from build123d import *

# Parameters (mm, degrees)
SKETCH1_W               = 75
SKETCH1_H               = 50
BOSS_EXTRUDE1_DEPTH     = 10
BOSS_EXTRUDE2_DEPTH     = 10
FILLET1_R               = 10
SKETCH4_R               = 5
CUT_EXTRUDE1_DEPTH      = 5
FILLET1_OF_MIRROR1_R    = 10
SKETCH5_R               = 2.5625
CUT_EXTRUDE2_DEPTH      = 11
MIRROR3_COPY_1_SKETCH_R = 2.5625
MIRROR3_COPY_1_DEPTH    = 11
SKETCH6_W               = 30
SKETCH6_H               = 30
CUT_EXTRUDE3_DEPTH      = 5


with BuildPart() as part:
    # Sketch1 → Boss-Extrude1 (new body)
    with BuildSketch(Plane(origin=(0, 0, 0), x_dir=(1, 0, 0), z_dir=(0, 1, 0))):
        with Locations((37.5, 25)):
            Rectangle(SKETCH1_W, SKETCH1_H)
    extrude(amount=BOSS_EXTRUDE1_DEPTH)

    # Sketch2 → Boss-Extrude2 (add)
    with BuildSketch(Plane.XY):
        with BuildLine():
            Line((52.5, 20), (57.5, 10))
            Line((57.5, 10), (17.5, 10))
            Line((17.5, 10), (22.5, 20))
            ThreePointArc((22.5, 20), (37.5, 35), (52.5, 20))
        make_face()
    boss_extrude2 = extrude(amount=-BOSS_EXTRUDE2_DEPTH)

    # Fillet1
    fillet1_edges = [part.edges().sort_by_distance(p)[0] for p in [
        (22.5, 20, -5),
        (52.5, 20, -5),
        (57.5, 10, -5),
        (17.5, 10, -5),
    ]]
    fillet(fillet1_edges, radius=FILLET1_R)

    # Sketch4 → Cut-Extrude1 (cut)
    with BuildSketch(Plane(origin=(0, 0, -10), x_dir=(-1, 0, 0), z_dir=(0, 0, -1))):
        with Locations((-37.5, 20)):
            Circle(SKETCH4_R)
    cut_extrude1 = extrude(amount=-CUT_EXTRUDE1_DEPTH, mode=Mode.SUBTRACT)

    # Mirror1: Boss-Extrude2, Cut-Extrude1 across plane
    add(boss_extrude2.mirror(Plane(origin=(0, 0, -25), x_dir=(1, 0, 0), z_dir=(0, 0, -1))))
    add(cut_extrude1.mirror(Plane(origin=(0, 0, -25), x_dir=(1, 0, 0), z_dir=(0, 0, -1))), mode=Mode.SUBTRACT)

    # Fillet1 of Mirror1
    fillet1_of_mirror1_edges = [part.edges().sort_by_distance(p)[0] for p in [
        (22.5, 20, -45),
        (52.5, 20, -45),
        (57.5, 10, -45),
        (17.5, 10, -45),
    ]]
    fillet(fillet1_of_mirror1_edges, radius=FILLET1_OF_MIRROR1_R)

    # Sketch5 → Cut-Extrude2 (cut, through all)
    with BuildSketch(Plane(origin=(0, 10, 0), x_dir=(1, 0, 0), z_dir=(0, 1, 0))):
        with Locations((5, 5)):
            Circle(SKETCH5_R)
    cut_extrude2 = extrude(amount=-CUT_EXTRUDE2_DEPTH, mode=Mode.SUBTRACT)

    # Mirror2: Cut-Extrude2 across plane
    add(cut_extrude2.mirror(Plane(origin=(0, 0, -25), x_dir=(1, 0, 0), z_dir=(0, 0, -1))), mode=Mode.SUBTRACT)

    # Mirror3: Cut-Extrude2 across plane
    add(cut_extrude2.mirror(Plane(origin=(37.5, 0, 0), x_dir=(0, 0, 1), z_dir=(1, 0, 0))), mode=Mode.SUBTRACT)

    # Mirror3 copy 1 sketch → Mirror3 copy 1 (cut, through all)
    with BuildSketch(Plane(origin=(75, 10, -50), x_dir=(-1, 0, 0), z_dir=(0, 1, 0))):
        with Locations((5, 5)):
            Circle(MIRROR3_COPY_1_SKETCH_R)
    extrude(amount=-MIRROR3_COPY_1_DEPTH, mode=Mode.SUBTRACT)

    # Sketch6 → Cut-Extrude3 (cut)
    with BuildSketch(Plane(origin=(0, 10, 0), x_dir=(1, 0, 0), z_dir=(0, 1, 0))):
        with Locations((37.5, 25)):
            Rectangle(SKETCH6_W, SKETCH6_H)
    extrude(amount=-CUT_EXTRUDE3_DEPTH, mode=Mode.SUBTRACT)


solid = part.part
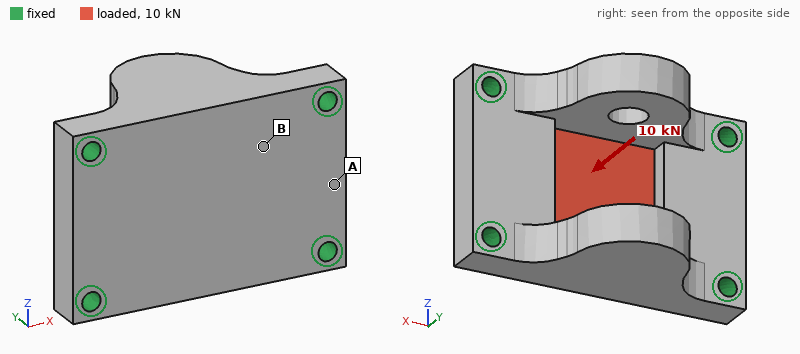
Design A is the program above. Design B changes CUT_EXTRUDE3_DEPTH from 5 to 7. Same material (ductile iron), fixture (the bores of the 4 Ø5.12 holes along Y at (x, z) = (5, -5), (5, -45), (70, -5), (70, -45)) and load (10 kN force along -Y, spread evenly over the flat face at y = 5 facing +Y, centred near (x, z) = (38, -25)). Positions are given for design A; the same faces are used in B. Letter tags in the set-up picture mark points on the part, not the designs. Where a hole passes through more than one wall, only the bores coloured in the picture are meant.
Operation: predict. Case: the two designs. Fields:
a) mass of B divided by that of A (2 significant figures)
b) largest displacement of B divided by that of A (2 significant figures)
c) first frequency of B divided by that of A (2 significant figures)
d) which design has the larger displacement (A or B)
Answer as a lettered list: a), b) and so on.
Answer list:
a) 0.96
b) 1.8
c) 0.98
d) B
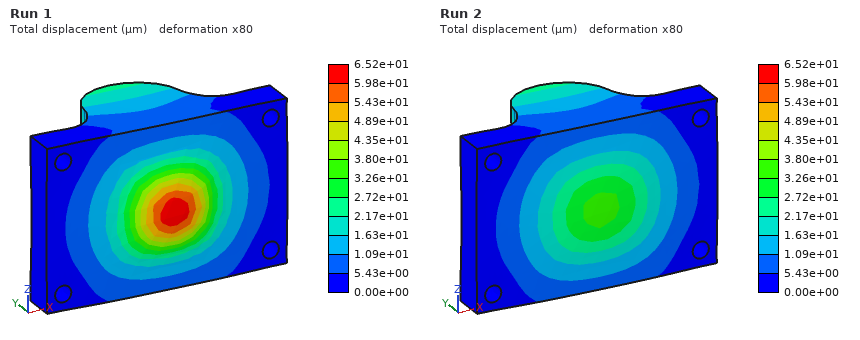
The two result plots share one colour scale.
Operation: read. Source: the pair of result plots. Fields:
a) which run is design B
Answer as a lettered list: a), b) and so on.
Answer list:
a) Run 1
